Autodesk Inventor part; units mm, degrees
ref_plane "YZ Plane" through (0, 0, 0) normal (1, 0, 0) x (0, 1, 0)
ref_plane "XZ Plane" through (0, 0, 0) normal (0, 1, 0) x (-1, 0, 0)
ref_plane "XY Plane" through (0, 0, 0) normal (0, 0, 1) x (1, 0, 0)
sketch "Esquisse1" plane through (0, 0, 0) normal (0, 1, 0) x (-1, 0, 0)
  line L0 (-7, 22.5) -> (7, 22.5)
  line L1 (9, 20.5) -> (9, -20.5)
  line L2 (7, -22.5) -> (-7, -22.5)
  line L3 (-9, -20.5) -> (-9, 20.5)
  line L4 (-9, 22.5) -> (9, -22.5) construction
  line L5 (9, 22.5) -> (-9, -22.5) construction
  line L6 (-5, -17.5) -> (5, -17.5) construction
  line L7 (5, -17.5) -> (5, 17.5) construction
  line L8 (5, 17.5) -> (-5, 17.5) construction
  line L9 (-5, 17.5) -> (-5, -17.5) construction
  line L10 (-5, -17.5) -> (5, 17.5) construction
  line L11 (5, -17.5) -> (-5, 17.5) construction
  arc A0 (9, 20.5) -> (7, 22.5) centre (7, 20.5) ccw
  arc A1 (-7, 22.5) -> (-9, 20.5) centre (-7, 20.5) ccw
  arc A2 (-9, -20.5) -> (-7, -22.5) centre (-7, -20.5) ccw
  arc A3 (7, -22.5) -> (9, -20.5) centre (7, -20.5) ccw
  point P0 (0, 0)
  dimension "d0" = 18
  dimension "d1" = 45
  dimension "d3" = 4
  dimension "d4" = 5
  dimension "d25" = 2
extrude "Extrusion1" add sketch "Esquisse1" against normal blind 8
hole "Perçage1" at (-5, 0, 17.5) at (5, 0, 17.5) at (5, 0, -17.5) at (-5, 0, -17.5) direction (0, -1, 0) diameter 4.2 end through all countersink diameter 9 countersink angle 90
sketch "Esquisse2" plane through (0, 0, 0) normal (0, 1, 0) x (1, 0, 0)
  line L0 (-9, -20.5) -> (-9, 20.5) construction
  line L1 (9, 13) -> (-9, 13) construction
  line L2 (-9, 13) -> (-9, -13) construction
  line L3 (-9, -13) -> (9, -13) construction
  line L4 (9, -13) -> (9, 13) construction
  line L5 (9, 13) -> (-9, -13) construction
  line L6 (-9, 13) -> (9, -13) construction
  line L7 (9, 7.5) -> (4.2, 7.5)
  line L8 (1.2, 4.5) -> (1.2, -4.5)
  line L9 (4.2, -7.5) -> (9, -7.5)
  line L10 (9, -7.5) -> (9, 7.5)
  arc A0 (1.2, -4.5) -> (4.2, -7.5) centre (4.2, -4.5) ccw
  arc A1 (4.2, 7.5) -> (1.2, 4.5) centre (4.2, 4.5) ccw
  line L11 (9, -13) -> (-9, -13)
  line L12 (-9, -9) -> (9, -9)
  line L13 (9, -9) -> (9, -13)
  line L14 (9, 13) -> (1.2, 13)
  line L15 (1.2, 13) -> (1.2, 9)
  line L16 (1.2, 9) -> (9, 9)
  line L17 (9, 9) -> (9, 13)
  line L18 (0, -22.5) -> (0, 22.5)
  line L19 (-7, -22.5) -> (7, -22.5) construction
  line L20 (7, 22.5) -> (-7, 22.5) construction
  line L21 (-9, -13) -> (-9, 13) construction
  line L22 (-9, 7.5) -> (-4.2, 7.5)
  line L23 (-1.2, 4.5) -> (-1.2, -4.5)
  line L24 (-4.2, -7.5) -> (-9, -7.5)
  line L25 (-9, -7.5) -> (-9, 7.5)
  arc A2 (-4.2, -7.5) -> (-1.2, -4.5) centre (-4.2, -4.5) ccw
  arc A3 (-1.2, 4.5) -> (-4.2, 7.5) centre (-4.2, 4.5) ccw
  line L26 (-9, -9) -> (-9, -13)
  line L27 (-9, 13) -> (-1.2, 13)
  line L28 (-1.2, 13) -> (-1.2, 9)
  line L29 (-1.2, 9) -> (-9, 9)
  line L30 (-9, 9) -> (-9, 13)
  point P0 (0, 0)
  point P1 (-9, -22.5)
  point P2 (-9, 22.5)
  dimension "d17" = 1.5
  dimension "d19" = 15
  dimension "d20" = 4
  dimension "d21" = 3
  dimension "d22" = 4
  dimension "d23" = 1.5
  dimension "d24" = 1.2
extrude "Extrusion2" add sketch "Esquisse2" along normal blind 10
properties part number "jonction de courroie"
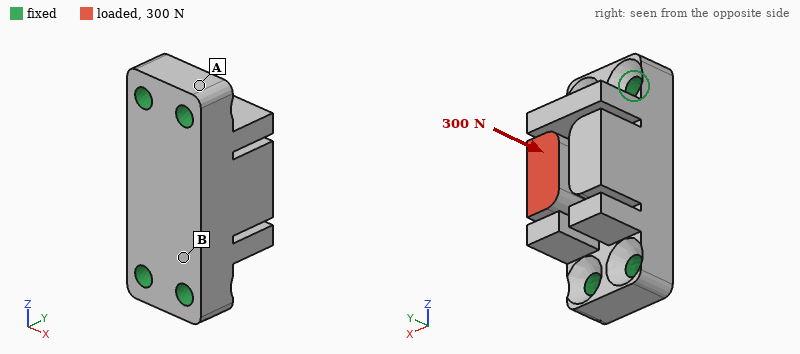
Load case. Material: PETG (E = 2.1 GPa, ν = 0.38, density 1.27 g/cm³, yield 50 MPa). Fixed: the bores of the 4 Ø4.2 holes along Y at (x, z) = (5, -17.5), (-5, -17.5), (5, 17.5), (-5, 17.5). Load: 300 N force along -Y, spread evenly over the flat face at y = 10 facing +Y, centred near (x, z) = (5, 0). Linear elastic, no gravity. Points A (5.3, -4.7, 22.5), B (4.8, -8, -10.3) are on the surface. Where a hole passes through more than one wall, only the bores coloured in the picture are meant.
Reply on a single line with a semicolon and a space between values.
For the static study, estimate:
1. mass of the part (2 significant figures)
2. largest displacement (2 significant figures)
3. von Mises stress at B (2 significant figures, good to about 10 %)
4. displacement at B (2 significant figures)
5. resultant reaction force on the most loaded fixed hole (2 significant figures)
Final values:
12 g; 0.10 mm; 2.9 MPa; 0.034 mm; 150 N
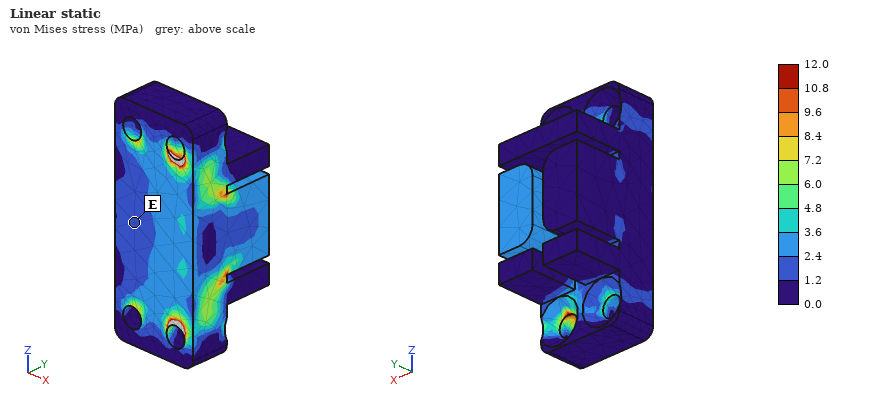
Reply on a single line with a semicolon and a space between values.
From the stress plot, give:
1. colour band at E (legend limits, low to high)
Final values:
1.2 to 2.4 MPa
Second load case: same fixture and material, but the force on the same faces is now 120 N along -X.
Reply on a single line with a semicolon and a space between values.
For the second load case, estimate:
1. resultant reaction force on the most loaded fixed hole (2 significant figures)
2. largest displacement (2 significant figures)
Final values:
92 N; 0.18 mm
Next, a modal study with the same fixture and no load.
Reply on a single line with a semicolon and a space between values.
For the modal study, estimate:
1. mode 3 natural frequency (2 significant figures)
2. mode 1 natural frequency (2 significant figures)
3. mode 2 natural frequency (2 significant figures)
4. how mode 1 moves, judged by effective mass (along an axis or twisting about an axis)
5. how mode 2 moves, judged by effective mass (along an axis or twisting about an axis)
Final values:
5900 Hz; 3900 Hz; 4600 Hz; along X; along Y
